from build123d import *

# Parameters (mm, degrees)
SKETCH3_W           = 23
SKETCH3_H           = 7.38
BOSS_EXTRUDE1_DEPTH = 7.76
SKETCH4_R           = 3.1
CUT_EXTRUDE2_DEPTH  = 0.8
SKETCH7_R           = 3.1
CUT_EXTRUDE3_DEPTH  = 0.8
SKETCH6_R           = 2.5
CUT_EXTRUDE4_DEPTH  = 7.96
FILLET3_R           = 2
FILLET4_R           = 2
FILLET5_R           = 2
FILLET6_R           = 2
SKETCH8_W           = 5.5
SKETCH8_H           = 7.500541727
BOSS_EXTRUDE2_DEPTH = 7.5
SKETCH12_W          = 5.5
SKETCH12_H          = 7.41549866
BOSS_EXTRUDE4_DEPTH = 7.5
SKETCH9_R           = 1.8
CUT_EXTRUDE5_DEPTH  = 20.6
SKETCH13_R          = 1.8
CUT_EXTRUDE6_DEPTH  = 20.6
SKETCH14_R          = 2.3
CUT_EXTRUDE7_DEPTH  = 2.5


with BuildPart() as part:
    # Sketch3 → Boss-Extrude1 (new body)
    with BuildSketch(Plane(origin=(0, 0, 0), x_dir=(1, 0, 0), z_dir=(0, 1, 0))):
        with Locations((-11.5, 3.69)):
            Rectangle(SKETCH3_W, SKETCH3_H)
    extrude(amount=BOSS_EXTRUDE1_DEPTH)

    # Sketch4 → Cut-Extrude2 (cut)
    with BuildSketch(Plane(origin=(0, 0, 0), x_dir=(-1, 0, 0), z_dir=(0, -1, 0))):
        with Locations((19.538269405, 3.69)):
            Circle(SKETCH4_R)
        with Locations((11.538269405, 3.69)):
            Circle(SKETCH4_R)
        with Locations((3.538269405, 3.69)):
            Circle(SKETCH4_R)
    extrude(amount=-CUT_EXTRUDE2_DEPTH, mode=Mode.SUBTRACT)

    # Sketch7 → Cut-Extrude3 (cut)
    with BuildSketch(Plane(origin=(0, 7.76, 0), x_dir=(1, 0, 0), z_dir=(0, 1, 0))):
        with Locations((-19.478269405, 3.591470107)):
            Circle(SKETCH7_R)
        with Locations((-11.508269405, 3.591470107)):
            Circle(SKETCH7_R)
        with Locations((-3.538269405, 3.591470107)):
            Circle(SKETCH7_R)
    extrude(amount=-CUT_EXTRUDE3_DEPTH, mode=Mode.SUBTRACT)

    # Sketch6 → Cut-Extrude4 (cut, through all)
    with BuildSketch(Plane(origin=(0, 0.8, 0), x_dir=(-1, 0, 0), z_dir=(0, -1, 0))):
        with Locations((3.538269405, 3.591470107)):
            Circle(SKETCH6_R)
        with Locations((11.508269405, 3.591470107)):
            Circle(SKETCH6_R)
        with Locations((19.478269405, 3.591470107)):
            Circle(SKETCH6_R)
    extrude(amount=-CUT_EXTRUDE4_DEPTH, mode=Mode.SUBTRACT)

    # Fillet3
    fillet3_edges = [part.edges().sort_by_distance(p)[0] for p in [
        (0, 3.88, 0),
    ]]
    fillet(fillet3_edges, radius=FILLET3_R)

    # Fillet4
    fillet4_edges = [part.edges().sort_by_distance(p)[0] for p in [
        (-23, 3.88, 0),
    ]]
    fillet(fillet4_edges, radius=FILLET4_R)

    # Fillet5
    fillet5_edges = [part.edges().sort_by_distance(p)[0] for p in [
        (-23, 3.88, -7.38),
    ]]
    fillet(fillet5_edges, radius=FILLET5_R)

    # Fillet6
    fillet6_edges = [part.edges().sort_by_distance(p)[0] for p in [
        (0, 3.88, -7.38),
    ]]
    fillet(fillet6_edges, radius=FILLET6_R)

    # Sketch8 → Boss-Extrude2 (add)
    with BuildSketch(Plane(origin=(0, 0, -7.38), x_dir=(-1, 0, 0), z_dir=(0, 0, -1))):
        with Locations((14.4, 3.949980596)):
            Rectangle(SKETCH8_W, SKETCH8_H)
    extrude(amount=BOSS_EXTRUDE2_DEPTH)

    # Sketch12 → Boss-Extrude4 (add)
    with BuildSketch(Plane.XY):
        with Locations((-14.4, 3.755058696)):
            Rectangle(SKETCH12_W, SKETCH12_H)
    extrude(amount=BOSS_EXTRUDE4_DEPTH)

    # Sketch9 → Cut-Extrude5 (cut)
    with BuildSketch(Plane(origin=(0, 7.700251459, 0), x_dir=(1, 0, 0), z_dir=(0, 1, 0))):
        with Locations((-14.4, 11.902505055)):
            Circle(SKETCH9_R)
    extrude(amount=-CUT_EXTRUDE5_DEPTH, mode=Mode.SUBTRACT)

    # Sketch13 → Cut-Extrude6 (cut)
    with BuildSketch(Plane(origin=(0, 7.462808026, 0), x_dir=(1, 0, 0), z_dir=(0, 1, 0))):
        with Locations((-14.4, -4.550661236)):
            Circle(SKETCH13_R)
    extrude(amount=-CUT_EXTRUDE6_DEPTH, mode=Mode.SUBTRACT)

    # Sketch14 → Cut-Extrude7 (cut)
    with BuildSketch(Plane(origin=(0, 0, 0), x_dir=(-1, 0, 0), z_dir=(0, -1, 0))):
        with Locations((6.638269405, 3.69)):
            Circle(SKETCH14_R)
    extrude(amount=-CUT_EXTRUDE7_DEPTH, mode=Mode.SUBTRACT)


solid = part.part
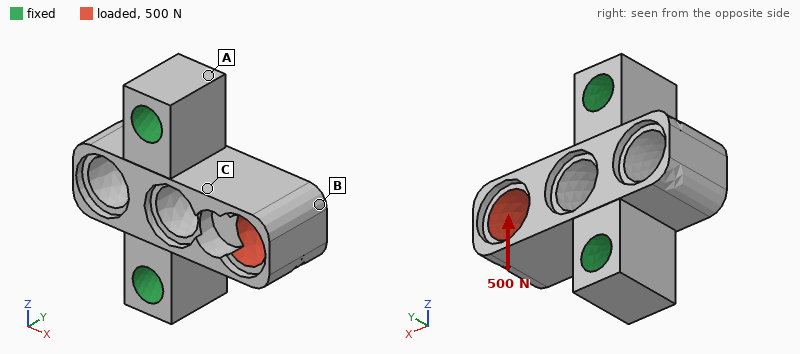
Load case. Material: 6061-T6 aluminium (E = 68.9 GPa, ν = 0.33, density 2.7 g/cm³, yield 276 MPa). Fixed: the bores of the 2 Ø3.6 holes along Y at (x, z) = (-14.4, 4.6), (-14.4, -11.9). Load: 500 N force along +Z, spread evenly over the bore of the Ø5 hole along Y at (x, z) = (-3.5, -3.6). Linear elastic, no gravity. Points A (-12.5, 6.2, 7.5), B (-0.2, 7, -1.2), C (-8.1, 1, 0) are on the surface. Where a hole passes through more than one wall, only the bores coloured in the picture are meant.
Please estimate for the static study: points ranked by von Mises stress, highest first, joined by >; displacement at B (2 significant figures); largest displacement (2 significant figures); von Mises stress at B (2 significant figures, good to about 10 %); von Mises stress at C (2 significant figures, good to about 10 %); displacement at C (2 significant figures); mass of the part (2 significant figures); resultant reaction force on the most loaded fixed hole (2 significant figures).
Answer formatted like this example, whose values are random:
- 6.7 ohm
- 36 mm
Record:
- C > B > A
- 41 µm
- 52 µm
- 27 MPa
- 45 MPa
- 14 µm
- 3.3 g
- 510 N
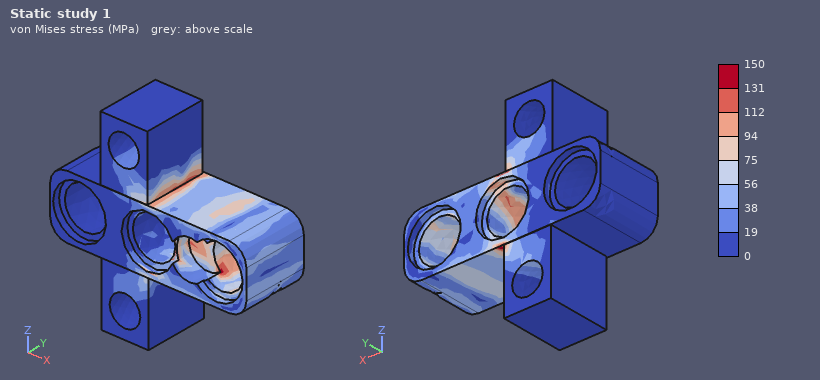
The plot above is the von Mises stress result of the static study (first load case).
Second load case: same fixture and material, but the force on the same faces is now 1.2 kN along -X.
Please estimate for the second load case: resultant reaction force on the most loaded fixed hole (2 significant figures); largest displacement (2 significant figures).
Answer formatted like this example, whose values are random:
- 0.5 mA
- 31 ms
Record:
- 610 N
- 18 µm
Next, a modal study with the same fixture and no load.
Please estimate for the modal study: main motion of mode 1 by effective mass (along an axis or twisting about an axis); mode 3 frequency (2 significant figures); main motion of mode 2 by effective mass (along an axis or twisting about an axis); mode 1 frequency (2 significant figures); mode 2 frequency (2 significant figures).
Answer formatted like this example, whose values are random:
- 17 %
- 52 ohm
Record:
- along Y
- 34 kHz
- along Z
- 19 kHz
- 24 kHz
